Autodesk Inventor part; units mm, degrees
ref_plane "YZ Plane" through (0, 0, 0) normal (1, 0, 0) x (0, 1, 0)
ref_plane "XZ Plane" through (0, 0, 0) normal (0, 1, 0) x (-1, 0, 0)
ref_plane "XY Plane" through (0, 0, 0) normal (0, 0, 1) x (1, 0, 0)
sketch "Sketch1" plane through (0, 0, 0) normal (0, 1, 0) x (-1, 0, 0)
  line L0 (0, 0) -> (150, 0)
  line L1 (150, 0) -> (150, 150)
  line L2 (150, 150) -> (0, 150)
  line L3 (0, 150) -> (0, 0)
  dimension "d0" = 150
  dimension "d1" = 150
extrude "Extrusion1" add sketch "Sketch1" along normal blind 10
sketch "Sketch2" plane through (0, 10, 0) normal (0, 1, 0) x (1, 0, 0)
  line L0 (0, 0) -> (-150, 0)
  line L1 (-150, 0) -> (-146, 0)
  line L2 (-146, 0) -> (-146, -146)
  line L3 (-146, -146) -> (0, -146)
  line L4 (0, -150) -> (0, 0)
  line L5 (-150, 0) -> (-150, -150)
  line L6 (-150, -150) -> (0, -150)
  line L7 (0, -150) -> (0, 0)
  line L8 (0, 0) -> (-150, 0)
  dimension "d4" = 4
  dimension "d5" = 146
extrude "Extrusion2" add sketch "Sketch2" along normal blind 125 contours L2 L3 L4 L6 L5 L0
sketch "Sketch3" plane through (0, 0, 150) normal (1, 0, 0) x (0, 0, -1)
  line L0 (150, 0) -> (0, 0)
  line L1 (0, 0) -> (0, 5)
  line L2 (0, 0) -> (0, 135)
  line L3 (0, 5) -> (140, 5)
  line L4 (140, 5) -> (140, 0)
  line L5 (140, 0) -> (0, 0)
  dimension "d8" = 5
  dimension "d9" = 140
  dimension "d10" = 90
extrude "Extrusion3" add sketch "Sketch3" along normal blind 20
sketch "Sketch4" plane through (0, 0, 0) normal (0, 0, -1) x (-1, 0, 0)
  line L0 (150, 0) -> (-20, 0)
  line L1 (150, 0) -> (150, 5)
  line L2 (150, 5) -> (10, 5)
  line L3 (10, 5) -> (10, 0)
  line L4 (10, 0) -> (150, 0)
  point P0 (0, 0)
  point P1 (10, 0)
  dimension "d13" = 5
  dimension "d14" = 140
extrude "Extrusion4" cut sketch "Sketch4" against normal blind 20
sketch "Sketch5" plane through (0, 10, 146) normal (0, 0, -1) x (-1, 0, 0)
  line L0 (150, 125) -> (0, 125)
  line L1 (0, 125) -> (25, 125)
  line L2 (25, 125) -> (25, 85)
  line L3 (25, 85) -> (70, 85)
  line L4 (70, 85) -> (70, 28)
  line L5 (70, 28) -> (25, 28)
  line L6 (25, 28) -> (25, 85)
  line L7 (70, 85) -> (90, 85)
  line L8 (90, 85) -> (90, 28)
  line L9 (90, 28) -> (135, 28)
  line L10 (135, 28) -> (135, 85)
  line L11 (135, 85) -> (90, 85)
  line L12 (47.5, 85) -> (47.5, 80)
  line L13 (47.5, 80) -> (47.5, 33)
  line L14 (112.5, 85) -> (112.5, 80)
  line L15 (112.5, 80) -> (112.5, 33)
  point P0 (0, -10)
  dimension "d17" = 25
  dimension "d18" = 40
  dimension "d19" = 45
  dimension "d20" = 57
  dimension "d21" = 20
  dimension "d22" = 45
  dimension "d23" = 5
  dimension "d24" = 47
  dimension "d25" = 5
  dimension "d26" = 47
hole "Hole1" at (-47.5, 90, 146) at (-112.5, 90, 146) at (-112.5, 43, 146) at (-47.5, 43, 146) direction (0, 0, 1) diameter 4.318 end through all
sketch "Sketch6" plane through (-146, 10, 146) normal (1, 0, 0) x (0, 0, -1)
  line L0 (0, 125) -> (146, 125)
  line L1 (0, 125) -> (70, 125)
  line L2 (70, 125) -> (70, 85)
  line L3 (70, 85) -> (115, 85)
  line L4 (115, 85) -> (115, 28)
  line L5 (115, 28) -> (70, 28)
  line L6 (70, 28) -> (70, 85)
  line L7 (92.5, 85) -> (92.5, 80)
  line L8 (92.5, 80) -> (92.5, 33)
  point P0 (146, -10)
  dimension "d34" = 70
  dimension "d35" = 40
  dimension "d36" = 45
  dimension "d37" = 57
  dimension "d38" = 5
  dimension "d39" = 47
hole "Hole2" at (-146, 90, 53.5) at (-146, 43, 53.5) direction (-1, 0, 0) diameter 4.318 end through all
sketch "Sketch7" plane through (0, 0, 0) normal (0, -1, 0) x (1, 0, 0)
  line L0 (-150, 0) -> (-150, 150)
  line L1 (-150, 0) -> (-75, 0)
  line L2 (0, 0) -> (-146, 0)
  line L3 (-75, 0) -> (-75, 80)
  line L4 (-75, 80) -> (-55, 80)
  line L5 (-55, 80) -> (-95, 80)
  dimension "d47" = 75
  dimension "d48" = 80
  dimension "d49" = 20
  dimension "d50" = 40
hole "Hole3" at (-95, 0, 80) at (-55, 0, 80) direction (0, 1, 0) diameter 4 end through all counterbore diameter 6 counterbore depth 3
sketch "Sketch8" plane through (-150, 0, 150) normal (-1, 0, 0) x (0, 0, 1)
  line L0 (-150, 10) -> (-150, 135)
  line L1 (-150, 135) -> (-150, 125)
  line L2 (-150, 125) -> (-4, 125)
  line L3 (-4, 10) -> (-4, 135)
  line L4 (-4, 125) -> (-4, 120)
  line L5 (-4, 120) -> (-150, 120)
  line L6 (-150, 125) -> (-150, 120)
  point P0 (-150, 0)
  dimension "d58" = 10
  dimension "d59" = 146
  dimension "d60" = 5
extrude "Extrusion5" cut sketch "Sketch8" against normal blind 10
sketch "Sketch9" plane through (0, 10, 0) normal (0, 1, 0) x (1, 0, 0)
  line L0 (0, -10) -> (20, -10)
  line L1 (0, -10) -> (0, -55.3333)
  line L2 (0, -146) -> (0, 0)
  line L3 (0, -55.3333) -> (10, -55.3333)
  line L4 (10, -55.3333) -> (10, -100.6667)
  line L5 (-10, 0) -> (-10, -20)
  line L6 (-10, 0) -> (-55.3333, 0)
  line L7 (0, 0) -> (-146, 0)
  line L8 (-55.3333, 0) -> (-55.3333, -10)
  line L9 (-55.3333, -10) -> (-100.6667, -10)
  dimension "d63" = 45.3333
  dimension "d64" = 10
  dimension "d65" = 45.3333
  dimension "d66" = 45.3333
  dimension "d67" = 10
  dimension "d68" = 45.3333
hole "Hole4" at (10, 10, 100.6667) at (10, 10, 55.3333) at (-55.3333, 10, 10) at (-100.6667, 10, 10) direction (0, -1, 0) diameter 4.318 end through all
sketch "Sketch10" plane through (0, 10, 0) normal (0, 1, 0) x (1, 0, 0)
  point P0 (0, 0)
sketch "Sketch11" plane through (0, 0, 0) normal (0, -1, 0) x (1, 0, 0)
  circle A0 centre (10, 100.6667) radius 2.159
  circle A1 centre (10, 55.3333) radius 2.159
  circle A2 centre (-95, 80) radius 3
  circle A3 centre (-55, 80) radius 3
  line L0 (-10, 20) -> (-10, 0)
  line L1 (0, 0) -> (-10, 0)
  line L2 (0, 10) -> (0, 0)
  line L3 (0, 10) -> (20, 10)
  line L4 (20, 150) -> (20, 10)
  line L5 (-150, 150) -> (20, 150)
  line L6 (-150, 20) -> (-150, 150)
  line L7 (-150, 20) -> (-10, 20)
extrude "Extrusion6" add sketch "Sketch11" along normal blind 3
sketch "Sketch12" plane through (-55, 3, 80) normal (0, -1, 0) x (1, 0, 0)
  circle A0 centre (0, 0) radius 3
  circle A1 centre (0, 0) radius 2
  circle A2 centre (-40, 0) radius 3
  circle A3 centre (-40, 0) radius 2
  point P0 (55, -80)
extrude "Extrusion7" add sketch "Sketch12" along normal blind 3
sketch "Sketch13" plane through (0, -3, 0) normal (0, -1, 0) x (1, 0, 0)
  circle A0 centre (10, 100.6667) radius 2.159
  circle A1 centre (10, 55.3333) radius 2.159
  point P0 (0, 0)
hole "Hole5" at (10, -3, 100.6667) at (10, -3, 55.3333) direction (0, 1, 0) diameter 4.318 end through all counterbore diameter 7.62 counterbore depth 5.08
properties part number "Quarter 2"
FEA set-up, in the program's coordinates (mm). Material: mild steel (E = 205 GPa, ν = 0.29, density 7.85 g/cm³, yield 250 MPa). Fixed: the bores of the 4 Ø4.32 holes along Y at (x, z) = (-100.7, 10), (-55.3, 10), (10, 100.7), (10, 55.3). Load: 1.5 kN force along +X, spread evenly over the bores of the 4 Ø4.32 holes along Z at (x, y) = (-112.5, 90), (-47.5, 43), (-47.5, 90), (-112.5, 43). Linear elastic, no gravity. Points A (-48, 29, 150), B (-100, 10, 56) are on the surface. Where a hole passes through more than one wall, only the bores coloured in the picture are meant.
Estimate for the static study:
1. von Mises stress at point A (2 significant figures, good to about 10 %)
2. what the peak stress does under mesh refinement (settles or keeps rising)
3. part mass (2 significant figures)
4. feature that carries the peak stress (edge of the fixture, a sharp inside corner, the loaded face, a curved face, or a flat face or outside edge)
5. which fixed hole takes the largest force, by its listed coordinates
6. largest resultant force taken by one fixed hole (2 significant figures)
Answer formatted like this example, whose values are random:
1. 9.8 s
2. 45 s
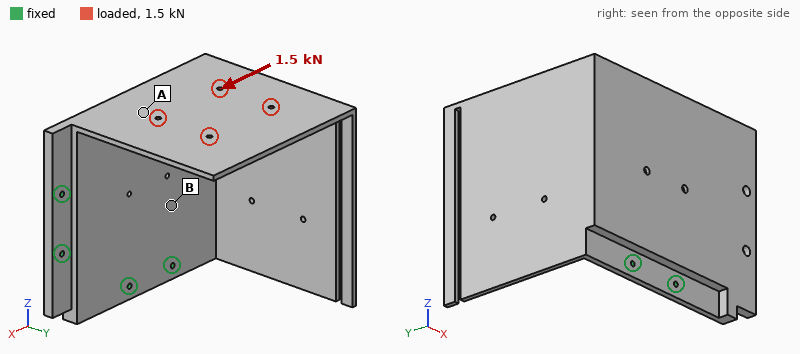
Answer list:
1. 5.9 MPa
2. keeps rising
3. 3.4 kg
4. edge of the fixture
5. (10, 100.7)
6. 2.3 kN
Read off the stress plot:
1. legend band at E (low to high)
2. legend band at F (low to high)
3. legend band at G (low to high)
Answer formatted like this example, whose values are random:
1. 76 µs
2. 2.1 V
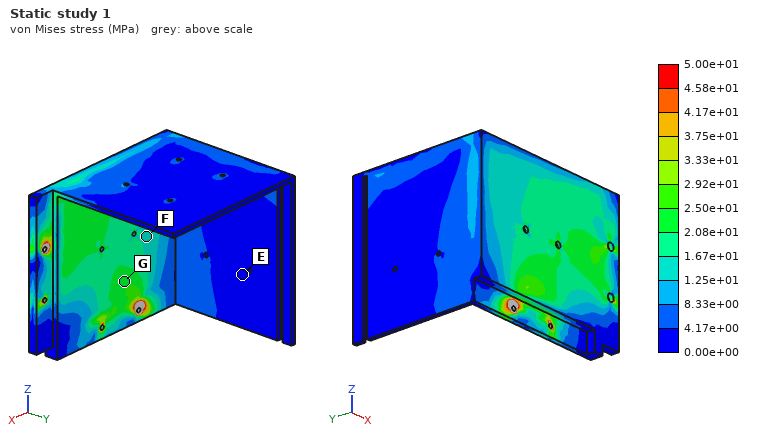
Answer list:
1. 0.00e+00 to 4.17e+00 MPa
2. 1.25e+01 to 1.67e+01 MPa
3. 2.08e+01 to 2.50e+01 MPa
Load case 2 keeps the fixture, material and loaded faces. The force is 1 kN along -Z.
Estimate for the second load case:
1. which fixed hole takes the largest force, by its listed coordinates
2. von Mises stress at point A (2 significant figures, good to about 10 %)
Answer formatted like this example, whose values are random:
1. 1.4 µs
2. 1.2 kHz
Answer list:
1. (10, 100.7)
2. 43 MPa
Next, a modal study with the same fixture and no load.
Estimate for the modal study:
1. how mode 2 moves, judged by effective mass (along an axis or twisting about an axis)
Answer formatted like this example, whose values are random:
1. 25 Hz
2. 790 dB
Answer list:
1. along Y
